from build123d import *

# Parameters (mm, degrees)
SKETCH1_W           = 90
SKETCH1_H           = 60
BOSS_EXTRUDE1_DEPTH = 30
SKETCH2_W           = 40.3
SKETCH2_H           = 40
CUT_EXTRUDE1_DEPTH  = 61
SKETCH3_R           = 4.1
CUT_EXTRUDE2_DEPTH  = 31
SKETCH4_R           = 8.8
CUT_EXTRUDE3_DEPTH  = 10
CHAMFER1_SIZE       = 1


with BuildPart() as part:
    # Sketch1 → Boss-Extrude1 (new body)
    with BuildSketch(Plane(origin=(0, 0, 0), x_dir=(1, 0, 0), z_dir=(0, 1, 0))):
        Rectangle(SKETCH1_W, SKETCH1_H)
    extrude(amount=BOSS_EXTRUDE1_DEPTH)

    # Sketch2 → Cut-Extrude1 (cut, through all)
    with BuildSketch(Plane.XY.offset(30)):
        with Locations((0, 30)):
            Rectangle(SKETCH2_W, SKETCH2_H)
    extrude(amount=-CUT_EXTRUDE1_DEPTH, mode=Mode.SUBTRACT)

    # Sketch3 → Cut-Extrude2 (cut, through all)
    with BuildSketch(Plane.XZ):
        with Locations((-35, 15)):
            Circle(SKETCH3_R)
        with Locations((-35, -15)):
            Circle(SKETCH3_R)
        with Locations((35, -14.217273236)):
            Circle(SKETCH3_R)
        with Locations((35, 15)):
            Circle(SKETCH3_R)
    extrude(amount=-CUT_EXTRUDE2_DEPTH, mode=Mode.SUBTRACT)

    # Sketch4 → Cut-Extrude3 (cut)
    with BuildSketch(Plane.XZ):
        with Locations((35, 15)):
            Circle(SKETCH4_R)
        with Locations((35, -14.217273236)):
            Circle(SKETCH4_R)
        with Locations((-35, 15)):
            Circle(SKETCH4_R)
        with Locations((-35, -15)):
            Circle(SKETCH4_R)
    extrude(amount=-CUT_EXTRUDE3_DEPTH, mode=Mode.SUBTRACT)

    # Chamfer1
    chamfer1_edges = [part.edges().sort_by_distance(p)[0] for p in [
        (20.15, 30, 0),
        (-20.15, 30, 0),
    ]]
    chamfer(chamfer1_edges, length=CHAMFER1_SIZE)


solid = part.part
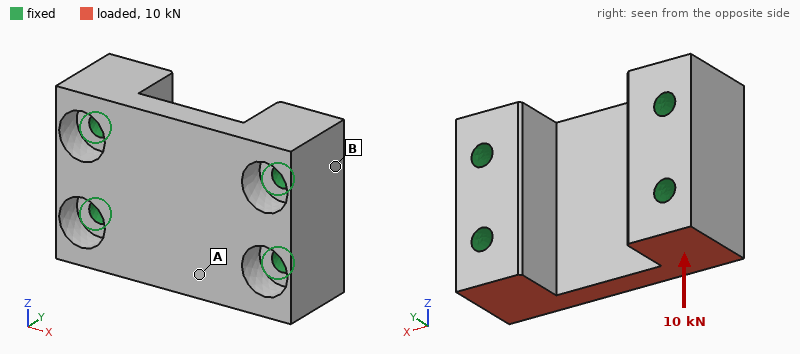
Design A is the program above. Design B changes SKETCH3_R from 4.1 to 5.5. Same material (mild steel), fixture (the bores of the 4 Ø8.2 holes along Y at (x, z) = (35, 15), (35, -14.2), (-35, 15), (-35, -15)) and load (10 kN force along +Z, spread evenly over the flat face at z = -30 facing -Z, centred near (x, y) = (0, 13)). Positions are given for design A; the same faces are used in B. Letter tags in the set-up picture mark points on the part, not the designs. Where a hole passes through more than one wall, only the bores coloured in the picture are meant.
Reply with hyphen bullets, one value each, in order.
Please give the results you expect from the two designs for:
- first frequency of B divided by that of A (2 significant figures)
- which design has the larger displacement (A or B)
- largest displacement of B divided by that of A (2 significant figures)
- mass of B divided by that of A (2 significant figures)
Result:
- 1.0
- A
- 0.91
- 0.97
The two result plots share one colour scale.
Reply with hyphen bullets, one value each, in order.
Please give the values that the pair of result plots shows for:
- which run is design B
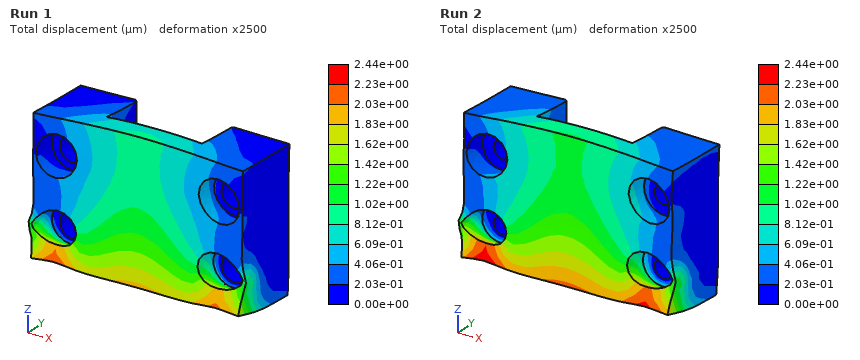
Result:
- Run 1
